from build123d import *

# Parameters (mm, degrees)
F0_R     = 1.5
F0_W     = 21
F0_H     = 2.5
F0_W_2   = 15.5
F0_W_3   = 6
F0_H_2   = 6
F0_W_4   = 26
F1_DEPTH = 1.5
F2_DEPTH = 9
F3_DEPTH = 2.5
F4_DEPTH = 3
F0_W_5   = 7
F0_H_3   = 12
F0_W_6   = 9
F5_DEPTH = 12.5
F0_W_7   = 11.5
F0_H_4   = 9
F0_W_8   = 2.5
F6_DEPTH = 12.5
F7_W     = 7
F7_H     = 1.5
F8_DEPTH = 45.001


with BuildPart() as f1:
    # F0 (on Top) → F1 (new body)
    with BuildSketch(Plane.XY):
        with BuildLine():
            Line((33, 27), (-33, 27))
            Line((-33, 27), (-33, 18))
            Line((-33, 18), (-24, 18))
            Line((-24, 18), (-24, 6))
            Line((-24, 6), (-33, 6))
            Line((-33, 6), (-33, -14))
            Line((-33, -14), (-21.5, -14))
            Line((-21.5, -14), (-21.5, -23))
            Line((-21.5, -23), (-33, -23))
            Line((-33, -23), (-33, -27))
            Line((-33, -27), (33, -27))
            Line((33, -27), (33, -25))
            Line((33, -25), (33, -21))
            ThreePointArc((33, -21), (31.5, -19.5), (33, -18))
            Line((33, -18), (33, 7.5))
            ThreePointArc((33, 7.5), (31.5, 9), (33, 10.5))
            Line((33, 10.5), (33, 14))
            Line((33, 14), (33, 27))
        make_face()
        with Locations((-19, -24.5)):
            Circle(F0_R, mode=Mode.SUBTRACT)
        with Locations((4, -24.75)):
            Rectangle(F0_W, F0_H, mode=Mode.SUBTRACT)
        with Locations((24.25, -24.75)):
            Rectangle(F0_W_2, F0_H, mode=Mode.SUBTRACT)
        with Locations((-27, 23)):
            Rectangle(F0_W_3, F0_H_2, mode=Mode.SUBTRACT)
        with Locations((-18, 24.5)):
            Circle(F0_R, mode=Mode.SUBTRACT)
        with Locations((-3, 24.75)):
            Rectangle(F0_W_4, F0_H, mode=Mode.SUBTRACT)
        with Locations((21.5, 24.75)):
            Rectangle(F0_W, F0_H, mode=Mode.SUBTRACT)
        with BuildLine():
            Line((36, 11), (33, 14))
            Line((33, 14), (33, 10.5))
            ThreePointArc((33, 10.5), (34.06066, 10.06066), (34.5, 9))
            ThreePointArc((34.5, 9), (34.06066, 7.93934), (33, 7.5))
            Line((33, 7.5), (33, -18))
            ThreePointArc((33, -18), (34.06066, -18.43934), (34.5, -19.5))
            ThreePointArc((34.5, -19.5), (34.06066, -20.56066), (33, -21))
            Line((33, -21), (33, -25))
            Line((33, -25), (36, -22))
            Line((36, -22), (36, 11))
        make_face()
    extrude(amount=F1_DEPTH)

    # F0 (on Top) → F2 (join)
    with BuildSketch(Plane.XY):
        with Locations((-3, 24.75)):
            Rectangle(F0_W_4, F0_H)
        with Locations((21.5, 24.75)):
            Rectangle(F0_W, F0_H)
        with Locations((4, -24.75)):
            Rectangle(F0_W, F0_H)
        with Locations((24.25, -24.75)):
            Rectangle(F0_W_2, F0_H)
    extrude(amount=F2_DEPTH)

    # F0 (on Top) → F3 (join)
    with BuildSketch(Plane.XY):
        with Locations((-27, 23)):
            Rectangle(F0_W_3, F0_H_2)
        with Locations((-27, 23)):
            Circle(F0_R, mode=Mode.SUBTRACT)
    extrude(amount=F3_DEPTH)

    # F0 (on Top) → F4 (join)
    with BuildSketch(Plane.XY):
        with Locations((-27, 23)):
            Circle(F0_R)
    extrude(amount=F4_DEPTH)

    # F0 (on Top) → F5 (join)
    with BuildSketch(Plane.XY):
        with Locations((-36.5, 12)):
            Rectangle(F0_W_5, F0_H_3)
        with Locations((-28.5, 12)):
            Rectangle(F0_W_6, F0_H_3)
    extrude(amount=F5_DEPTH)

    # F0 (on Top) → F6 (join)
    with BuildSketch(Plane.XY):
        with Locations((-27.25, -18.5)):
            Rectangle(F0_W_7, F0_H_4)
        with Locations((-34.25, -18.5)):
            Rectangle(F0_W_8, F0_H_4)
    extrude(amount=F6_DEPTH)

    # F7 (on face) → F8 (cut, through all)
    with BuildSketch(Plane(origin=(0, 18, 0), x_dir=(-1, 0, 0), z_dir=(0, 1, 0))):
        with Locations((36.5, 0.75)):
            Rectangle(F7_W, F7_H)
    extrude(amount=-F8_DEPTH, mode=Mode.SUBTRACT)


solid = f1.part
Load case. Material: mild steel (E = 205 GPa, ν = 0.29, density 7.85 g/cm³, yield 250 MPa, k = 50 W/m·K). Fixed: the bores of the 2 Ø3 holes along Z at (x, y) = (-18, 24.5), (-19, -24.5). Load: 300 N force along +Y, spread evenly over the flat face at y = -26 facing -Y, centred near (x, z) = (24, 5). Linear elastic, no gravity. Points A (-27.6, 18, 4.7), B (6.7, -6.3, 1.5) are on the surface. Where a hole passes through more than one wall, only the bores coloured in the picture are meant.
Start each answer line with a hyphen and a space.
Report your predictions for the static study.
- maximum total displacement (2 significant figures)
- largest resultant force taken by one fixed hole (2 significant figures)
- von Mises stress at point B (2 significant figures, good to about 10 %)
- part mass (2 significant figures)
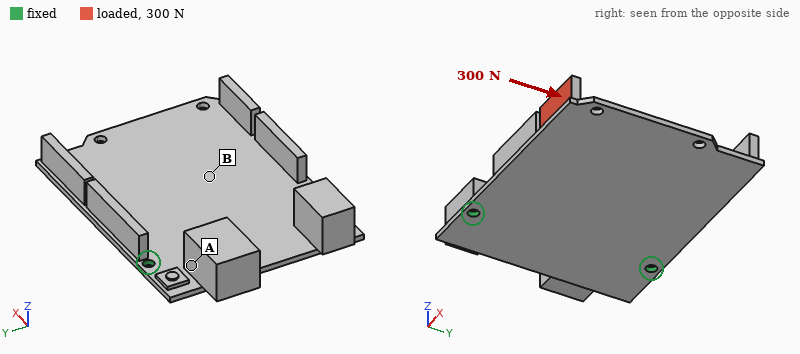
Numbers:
- 0.23 mm
- 310 N
- 49 MPa
- 83 g
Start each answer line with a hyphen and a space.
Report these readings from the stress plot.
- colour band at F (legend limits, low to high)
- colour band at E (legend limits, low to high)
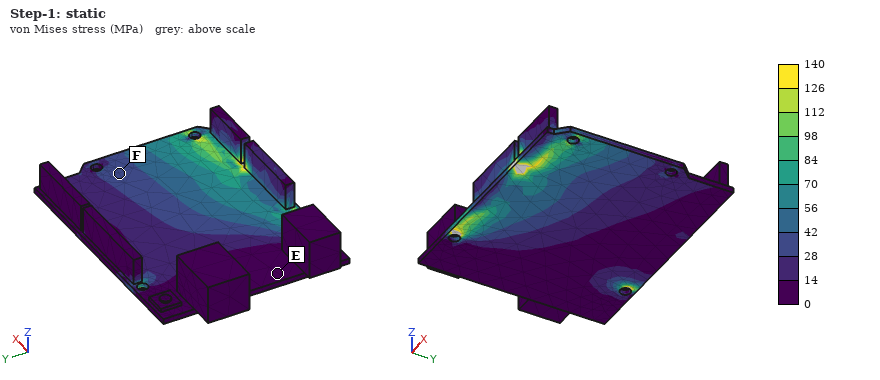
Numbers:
- 28 to 42 MPa
- 0 to 14 MPa
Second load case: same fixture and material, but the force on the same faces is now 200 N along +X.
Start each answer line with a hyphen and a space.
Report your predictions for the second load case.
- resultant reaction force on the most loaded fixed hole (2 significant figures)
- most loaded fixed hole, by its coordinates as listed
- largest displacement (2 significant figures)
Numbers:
- 210 N
- (-19, -24.5)
- 0.35 mm
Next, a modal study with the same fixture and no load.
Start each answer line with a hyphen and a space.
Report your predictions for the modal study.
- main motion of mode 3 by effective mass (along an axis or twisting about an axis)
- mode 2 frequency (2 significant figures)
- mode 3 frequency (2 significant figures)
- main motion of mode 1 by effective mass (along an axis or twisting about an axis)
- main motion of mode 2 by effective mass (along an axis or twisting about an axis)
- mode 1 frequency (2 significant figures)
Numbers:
- along Z
- 960 Hz
- 1100 Hz
- along Z
- twisting about X
- 420 Hz
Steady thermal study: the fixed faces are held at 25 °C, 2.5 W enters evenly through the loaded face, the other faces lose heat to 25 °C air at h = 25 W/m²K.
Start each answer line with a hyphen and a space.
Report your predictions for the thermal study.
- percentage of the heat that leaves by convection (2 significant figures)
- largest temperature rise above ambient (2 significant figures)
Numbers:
- 65 %
- 32 K
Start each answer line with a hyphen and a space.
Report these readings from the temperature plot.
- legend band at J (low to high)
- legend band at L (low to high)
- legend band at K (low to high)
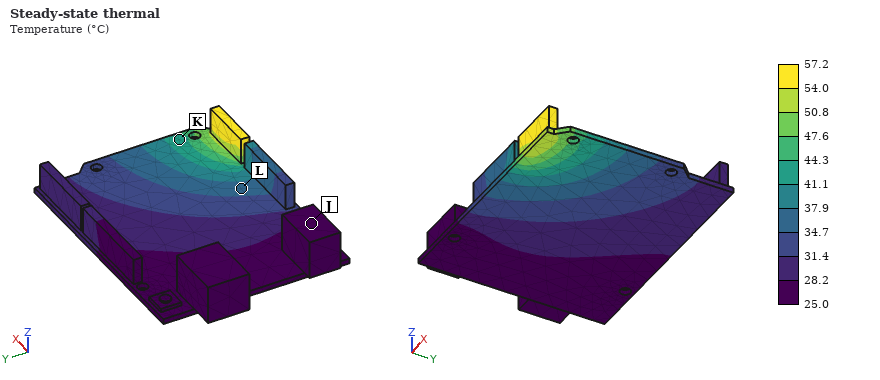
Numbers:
- 25.0 to 28.2 °C
- 34.7 to 37.9 °C
- 41.1 to 44.3 °C
